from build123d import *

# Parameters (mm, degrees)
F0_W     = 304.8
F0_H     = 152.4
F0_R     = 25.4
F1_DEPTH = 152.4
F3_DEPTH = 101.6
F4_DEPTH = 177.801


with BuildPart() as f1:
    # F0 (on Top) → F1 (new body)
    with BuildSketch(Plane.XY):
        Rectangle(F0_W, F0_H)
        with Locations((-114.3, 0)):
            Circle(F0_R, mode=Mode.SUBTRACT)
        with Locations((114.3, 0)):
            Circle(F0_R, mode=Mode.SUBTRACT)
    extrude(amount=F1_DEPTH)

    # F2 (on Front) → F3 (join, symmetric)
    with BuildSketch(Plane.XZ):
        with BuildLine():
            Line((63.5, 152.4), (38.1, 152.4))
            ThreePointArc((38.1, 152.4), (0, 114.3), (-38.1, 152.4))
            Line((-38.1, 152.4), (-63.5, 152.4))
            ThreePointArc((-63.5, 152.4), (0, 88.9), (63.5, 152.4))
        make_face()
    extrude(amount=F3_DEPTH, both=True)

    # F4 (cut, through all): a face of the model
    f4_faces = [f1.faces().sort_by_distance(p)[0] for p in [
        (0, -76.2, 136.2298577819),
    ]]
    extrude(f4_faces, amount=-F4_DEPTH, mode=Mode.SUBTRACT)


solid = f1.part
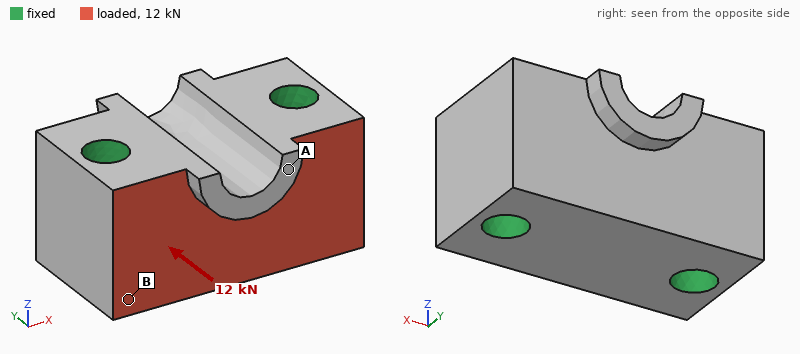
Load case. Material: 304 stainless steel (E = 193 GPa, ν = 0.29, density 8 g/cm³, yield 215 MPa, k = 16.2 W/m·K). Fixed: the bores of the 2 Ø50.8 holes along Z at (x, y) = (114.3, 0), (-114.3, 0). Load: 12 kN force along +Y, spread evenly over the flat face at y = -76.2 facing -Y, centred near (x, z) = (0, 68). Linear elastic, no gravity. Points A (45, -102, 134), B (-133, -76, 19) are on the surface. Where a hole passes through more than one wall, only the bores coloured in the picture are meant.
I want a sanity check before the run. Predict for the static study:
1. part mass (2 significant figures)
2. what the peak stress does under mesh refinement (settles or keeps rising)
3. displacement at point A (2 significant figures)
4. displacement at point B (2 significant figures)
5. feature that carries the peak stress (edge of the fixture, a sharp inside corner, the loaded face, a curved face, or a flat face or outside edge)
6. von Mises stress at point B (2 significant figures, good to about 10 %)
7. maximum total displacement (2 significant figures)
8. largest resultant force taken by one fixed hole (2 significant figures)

51 kg
keeps rising
0.13 µm
0.097 µm
edge of the fixture
0.33 MPa
0.31 µm
6.0 kN
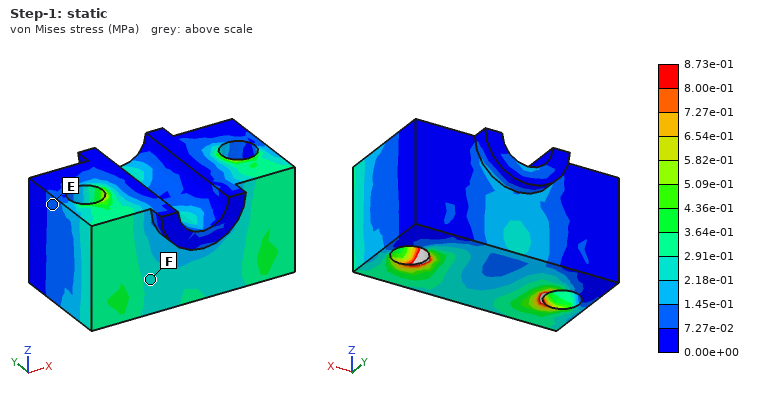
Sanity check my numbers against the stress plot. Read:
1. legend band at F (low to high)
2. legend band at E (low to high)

2.18e-01 to 2.91e-01 MPa
7.27e-02 to 1.45e-01 MPa
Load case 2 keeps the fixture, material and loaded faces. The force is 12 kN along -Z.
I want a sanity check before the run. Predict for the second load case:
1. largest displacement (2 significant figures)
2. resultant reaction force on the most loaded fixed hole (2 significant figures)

0.78 µm
6.0 kN
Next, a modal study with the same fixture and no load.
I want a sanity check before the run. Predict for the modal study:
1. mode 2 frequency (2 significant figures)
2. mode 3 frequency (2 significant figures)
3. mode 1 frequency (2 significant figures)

5900 Hz
6400 Hz
5700 Hz
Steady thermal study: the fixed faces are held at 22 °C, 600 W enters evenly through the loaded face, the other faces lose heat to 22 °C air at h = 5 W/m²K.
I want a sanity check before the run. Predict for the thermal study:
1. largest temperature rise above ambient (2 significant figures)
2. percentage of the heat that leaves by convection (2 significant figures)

78 K
3.0 %
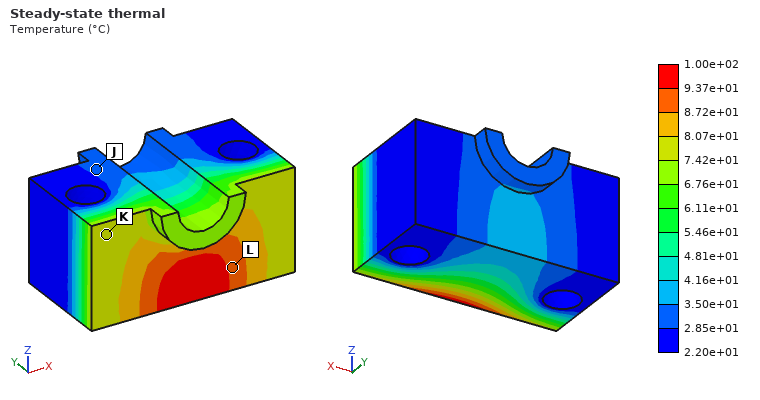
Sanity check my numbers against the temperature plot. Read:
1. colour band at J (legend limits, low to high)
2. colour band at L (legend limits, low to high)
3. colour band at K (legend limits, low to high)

2.85e+01 to 3.50e+01 °C
8.72e+01 to 9.37e+01 °C
7.42e+01 to 8.07e+01 °C
